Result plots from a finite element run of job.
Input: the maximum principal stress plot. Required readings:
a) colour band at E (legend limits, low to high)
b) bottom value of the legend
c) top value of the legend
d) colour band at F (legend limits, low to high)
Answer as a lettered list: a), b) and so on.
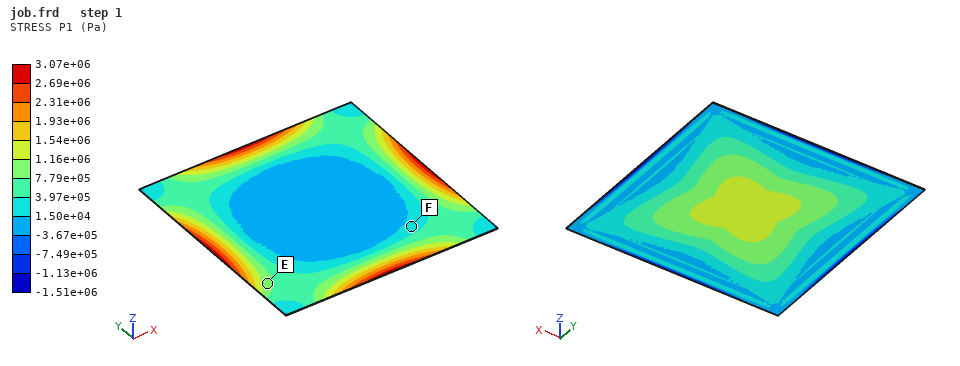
a) 7.79e+05 to 1.16e+06 Pa
b) -1.51e+06 Pa
c) 3.07e+06 Pa
d) 1.50e+04 to 3.97e+05 Pa
